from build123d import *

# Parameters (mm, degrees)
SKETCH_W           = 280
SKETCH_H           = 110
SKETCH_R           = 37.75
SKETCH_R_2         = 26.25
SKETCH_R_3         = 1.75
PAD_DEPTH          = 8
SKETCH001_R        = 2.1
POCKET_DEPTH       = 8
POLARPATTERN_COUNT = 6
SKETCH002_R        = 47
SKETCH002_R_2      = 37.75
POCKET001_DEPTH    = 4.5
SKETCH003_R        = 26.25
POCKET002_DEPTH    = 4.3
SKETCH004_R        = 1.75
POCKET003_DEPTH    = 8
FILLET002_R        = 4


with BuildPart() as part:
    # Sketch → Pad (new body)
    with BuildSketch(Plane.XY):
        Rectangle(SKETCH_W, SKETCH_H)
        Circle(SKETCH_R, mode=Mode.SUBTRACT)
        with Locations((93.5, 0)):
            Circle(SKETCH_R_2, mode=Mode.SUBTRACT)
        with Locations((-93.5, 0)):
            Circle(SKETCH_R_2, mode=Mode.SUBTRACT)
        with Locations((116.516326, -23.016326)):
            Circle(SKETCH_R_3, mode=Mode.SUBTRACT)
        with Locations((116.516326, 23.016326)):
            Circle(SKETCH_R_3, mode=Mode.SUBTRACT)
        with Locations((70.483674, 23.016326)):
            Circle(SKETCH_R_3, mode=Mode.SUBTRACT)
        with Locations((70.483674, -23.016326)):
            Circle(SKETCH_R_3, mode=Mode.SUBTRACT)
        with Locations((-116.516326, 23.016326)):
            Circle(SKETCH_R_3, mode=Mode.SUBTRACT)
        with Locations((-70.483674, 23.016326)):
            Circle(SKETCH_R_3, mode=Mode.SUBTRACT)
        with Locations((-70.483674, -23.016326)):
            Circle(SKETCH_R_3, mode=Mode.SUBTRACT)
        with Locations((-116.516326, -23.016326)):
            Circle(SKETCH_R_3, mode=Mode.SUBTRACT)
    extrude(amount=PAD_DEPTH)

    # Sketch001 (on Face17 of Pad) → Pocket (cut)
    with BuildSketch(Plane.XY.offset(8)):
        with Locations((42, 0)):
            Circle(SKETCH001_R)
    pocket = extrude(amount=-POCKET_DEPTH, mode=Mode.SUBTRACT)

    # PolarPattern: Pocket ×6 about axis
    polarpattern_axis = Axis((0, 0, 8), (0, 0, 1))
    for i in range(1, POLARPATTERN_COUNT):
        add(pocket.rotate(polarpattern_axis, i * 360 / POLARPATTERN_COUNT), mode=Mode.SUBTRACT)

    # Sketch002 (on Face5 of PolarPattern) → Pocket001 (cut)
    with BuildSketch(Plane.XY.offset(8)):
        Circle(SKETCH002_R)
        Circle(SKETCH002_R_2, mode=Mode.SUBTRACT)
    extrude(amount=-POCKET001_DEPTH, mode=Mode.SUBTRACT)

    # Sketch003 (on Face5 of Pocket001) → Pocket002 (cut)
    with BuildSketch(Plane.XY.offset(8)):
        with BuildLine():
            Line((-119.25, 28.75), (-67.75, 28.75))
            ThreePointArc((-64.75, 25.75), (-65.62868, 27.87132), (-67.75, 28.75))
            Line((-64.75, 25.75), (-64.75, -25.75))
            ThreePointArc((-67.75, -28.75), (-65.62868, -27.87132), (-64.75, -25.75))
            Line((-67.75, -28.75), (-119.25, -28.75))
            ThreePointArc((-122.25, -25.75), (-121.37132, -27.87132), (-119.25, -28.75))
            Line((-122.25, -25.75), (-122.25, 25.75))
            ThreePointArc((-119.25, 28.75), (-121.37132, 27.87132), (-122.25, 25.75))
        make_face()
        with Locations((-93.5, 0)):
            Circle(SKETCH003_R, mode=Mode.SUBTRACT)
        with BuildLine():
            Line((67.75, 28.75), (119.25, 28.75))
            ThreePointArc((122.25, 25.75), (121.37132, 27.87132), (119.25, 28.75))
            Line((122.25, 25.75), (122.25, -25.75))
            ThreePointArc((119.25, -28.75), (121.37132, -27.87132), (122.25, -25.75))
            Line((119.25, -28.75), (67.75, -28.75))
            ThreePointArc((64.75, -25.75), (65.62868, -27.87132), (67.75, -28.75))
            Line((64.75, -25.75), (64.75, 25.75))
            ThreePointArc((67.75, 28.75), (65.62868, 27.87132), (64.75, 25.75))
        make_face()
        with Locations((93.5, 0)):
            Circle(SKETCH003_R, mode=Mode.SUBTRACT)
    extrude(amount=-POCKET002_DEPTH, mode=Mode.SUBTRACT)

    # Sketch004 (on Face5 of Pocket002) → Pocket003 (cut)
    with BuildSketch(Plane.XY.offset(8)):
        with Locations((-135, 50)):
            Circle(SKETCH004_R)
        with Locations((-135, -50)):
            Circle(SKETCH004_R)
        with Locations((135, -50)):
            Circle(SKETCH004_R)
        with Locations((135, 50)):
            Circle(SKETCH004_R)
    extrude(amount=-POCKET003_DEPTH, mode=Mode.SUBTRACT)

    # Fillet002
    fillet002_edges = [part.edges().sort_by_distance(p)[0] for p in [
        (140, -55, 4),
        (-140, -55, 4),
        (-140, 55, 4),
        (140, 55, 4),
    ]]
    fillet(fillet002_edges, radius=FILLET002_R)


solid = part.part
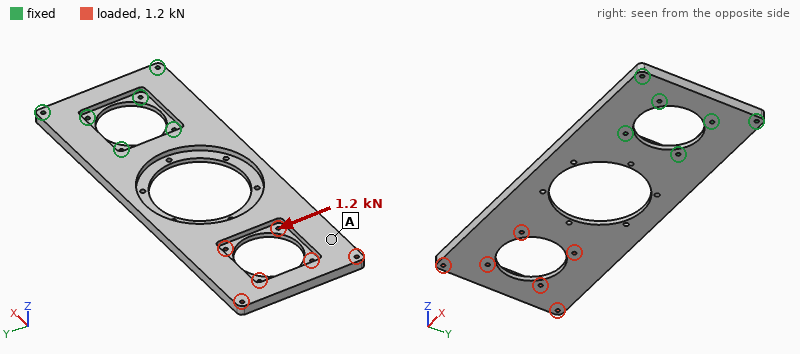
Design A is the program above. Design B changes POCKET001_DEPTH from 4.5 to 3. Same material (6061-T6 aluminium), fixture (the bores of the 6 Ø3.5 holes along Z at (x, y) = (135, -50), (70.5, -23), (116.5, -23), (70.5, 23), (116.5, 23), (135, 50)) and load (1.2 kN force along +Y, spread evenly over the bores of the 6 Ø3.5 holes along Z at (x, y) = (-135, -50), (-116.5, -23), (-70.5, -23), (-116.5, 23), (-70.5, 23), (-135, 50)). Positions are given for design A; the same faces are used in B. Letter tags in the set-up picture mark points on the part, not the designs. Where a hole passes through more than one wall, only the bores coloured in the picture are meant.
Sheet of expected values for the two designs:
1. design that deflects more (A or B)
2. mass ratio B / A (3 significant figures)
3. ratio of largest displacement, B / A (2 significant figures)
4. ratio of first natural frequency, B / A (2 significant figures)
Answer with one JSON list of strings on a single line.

["A", "1.02", "0.87", "1.0"]
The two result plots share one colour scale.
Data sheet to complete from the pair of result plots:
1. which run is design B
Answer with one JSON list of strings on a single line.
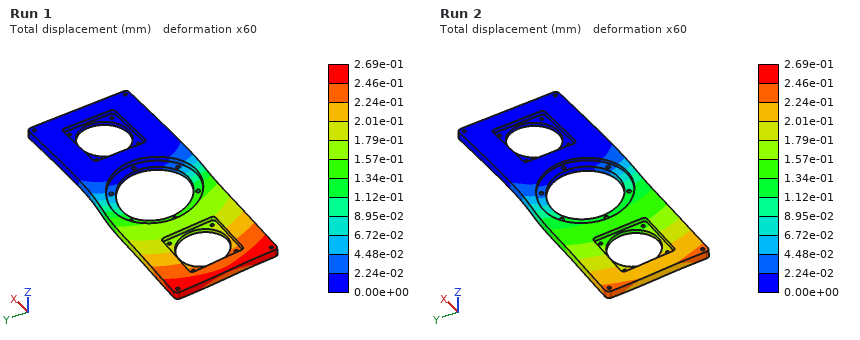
["Run 2"]
